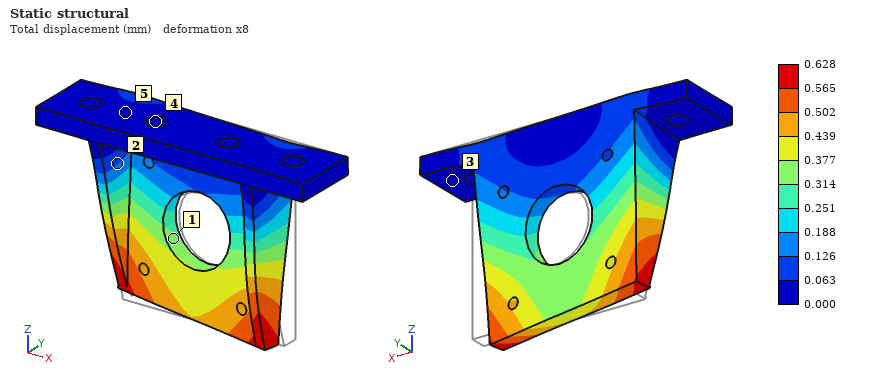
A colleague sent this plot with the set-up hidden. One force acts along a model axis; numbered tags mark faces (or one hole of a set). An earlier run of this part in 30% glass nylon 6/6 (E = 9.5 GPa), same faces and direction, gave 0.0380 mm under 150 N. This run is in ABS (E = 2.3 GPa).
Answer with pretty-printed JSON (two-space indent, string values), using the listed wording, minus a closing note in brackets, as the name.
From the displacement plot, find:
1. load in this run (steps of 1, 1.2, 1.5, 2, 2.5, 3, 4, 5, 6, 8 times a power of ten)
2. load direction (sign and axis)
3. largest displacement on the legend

{
  "load in this run": "600 N",
  "load direction": "-X",
  "largest displacement on the legend": "0.628 mm"
}
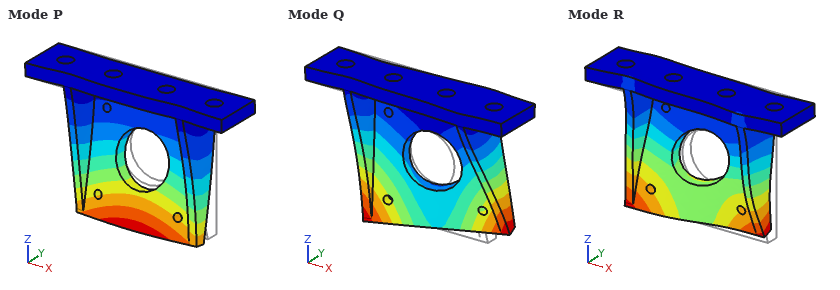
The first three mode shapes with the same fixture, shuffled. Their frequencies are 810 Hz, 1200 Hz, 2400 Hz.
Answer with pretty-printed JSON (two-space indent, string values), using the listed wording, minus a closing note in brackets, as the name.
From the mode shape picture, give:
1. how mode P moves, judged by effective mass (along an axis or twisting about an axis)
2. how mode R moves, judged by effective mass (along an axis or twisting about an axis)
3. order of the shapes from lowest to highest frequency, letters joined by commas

{
  "how mode P moves, judged by effective mass": "along Y",
  "how mode R moves, judged by effective mass": "along X",
  "order of the shapes from lowest to highest frequency, letters joined by commas": "P, Q, R"
}
